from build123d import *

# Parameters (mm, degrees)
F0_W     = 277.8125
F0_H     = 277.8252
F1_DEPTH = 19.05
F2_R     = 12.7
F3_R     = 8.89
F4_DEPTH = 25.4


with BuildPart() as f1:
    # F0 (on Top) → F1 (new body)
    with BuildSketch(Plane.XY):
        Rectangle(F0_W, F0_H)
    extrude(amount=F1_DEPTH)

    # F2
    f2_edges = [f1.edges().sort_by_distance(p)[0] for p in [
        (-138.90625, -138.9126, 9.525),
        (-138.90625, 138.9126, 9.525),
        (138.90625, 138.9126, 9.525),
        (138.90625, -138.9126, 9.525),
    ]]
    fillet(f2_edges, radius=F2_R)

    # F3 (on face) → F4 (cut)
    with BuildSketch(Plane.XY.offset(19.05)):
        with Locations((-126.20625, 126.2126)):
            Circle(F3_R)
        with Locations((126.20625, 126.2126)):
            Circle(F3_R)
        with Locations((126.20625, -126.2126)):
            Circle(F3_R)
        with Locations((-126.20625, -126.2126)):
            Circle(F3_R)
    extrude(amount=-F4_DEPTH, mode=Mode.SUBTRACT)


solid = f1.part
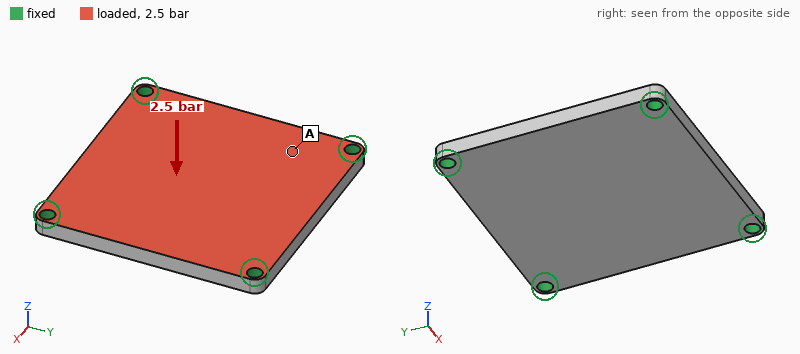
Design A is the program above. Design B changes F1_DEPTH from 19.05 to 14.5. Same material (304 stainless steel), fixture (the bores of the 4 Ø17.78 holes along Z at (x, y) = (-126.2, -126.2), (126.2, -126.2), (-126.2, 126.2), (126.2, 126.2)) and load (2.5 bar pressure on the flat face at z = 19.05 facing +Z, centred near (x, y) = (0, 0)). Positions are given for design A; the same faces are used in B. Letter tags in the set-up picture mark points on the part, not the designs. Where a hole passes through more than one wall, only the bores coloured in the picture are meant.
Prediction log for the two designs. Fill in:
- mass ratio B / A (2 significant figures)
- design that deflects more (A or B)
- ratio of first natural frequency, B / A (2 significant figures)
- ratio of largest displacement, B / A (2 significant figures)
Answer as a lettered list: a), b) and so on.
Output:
a) 0.76
b) B
c) 0.78
d) 2.2
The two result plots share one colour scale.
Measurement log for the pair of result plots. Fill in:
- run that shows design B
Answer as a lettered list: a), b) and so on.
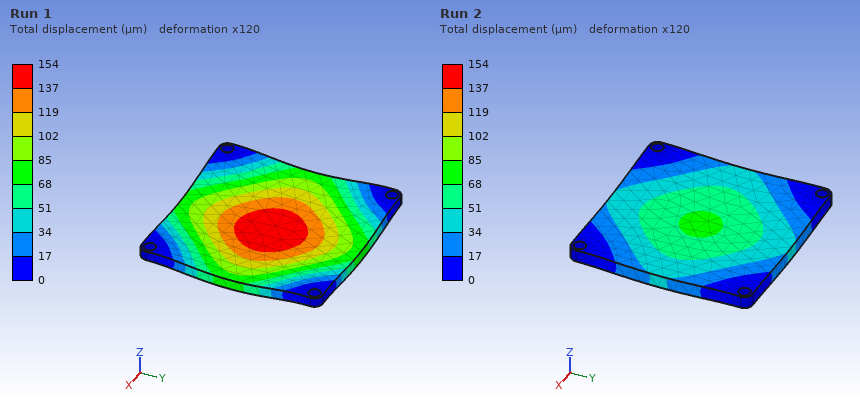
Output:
a) Run 1
